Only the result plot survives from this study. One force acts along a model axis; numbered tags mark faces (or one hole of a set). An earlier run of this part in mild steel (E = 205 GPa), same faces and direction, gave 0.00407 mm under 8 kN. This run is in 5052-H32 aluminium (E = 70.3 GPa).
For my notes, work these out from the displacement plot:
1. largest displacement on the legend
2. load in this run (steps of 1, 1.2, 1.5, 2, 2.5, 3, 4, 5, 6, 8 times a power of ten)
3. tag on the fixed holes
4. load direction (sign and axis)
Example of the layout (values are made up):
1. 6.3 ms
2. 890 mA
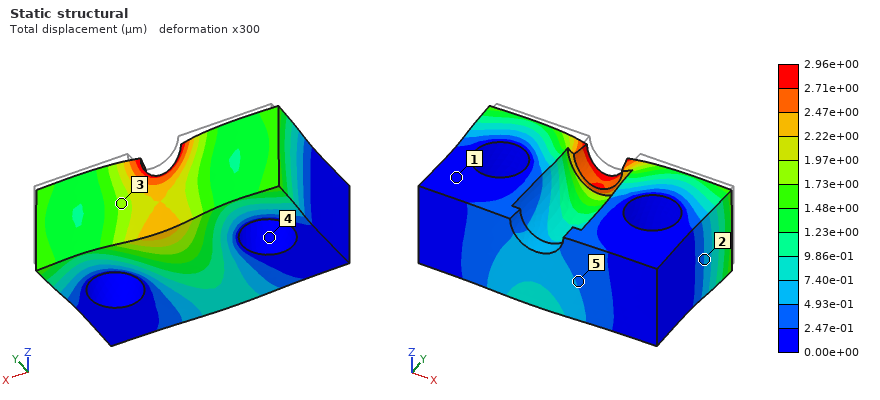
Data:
1. 2.96e+00 µm
2. 2 kN
3. 4
4. -Y
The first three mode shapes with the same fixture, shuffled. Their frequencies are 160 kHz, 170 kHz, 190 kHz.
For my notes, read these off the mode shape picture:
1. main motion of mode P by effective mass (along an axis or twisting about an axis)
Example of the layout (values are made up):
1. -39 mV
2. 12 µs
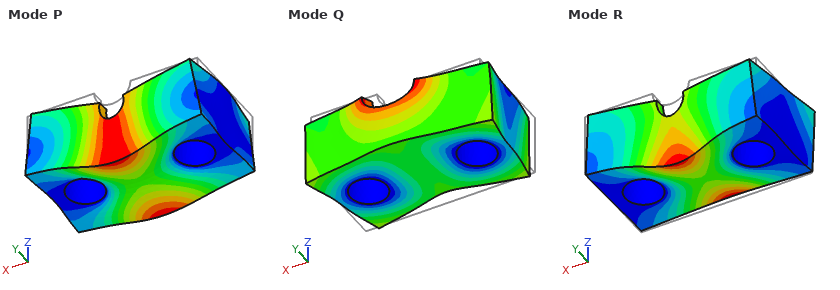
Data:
1. along Z
